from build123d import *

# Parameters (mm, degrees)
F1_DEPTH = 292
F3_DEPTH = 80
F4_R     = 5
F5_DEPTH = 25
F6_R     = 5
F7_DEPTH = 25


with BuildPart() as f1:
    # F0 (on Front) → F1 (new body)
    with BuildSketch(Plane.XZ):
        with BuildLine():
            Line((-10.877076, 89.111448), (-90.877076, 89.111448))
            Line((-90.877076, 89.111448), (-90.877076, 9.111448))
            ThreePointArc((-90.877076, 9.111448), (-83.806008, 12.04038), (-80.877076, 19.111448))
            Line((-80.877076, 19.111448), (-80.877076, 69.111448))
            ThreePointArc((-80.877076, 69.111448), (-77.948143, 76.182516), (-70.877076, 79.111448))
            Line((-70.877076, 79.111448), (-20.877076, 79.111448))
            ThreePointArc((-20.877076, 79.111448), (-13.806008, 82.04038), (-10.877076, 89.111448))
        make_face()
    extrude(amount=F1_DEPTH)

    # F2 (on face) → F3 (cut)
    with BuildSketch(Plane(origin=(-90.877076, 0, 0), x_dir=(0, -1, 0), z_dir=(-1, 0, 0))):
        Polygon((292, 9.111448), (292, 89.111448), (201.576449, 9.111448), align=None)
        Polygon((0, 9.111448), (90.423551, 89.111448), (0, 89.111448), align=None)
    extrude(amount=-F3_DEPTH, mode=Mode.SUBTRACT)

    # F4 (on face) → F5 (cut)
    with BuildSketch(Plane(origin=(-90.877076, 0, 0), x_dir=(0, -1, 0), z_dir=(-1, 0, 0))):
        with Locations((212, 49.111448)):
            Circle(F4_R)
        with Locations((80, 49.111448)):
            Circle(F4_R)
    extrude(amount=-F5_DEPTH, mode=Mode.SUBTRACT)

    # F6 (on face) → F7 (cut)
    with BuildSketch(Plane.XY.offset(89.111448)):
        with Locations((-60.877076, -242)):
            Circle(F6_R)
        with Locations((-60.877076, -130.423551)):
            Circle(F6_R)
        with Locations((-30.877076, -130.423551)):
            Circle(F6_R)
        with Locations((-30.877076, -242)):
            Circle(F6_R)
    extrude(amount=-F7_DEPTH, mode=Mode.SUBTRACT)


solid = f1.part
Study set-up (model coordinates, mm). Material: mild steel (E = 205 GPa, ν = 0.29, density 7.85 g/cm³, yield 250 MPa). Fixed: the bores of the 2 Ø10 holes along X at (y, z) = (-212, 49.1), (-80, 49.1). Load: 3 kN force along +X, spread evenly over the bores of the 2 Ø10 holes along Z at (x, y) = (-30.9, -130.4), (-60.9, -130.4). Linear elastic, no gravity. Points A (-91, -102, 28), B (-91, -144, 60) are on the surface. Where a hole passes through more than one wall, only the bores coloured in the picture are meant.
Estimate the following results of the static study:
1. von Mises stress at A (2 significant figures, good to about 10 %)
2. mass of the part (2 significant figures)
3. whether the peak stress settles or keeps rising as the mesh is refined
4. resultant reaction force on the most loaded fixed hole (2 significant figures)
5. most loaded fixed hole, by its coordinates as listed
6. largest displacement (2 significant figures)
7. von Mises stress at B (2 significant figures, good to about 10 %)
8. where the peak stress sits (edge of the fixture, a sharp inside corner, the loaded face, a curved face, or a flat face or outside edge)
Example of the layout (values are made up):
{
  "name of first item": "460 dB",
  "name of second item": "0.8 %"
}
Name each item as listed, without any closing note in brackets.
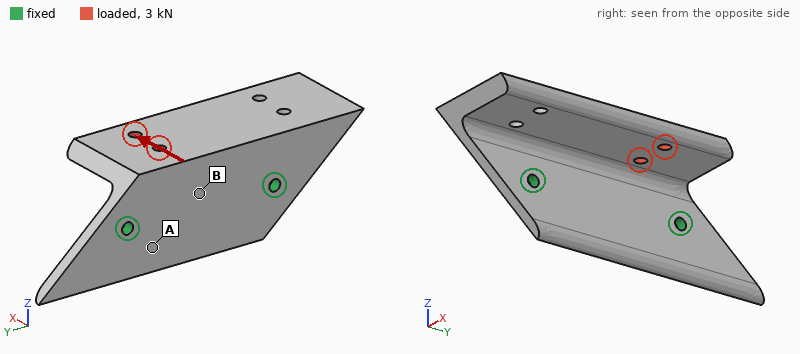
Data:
{
  "von Mises stress at A": "5.9 MPa",
  "mass of the part": "2.3 kg",
  "whether the peak stress settles or keeps rising as the mesh is refined": "keeps rising",
  "resultant reaction force on the most loaded fixed hole": "1.9 kN",
  "most loaded fixed hole, by its coordinates as listed": "(-80, 49.1)",
  "largest displacement": "80 µm",
  "von Mises stress at B": "9.4 MPa",
  "where the peak stress sits": "edge of the fixture"
}
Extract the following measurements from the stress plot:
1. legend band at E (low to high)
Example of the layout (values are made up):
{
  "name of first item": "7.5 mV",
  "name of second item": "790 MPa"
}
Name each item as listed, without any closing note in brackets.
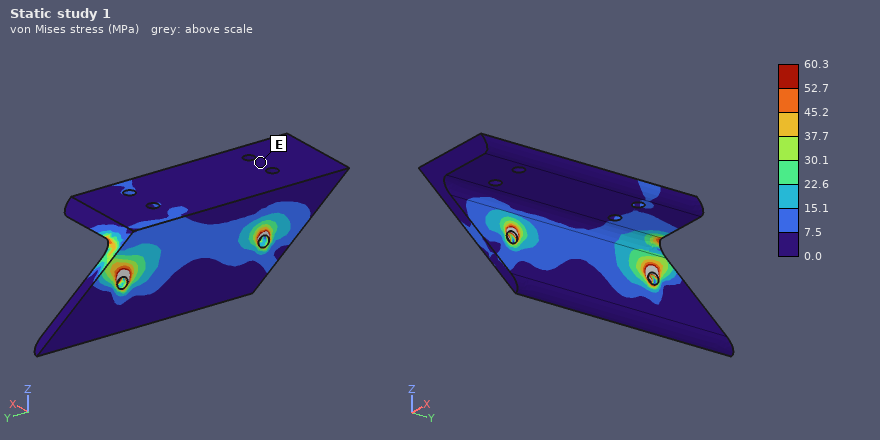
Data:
{
  "legend band at E": "0.0 to 7.5 MPa"
}
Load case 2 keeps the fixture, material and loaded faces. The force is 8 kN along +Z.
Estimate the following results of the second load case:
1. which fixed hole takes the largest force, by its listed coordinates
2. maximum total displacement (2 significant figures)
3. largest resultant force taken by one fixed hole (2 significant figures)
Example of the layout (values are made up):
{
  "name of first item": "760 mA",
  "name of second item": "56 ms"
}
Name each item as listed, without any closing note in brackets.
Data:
{
  "which fixed hole takes the largest force, by its listed coordinates": "(-80, 49.1)",
  "maximum total displacement": "0.50 mm",
  "largest resultant force taken by one fixed hole": "5.0 kN"
}
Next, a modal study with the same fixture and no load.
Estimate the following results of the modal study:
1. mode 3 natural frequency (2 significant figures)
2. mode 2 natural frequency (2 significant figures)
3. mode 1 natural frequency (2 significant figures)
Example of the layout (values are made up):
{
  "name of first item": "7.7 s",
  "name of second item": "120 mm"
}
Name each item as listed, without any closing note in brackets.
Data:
{
  "mode 3 natural frequency": "2000 Hz",
  "mode 2 natural frequency": "1400 Hz",
  "mode 1 natural frequency": "780 Hz"
}
